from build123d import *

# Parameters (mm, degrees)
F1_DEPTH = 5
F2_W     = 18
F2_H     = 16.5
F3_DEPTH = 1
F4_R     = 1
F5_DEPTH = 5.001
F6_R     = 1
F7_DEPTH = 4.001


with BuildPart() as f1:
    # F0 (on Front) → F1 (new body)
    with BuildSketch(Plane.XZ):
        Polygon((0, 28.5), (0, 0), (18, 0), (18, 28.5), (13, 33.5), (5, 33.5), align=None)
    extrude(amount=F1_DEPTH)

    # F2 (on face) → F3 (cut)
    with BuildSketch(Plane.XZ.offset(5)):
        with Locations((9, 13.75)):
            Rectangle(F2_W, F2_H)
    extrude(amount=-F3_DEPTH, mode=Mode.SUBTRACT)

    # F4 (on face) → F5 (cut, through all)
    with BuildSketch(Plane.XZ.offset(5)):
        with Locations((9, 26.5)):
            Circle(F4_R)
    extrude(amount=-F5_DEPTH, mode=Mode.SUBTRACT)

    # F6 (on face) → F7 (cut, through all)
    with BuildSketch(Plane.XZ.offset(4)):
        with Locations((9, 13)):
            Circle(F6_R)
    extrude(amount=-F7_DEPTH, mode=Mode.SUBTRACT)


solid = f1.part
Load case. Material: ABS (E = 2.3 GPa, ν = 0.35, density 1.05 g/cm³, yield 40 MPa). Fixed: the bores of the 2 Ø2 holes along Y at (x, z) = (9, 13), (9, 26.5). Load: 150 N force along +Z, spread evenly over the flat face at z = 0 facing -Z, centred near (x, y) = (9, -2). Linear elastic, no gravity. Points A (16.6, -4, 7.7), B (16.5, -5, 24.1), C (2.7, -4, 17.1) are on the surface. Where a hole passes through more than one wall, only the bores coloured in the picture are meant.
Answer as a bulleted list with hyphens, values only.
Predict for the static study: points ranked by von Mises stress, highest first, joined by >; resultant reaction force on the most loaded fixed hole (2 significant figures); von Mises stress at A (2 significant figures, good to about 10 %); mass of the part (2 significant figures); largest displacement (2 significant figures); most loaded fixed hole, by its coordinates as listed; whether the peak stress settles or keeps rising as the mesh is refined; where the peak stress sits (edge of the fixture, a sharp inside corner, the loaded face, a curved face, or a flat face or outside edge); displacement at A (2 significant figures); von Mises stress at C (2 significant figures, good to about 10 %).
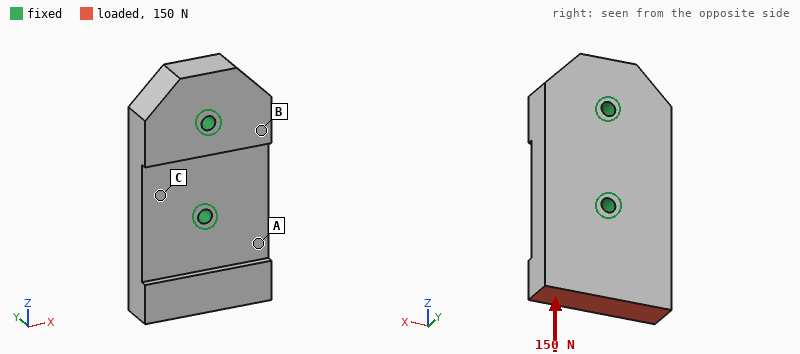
- A > C > B
- 110 N
- 3.0 MPa
- 2.7 g
- 40 µm
- (9, 13)
- keeps rising
- edge of the fixture
- 17 µm
- 1.5 MPa
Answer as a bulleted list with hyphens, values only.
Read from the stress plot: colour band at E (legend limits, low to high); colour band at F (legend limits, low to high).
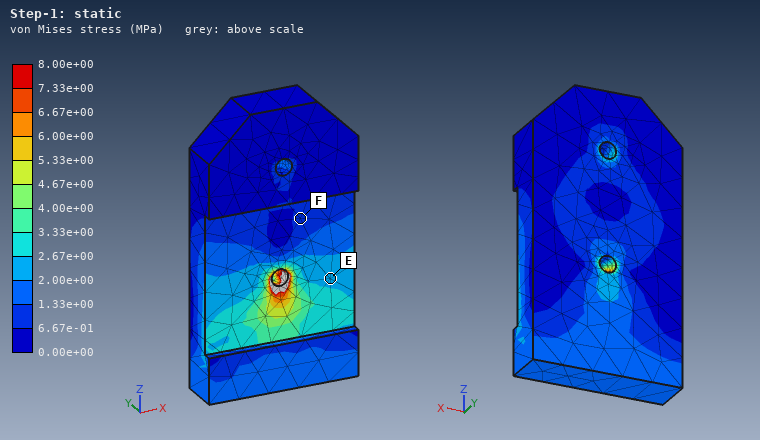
- 2.00e+00 to 2.67e+00 MPa
- 6.67e-01 to 1.33e+00 MPa
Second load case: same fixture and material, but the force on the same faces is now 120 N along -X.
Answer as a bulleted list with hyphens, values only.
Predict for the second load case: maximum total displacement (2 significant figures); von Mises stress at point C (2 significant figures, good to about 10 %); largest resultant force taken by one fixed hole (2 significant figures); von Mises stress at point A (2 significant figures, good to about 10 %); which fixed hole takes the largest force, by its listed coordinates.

- 0.12 mm
- 3.9 MPa
- 220 N
- 4.9 MPa
- (9, 13)
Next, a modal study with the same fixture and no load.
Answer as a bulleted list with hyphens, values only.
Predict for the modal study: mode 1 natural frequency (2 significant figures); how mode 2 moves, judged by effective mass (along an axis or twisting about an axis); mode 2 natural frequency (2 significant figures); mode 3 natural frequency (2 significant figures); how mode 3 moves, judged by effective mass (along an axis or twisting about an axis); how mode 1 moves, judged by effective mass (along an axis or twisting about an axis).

- 4100 Hz
- twisting about Z
- 5500 Hz
- 7600 Hz
- along X
- along Y
